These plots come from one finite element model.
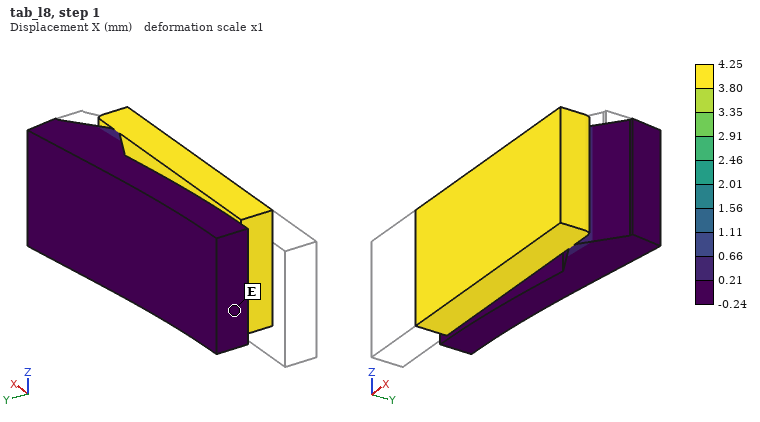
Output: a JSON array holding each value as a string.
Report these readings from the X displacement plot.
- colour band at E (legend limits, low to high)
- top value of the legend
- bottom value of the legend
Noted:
["-0.24 to 0.21 mm", "4.25 mm", "-0.24 mm"]
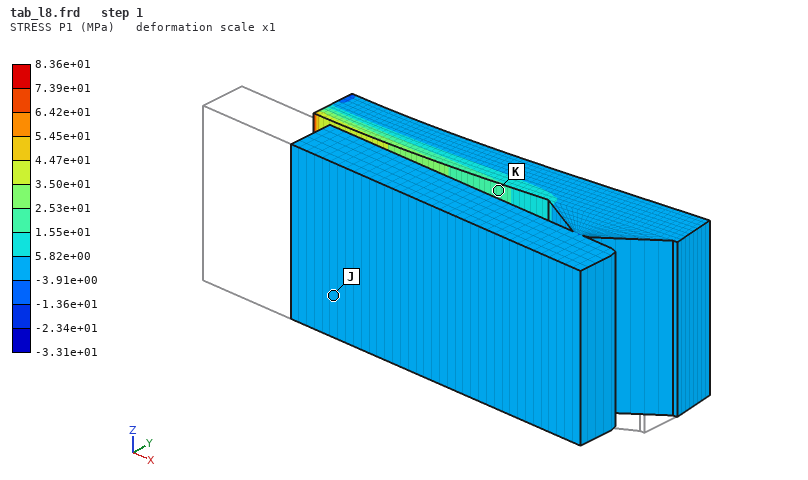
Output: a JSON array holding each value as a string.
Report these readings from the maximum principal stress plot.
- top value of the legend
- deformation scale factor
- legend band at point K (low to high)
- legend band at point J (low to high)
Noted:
["8.36e+01 MPa", "1", "1.55e+01 to 2.53e+01 MPa", "-3.91e+00 to 5.82e+00 MPa"]
